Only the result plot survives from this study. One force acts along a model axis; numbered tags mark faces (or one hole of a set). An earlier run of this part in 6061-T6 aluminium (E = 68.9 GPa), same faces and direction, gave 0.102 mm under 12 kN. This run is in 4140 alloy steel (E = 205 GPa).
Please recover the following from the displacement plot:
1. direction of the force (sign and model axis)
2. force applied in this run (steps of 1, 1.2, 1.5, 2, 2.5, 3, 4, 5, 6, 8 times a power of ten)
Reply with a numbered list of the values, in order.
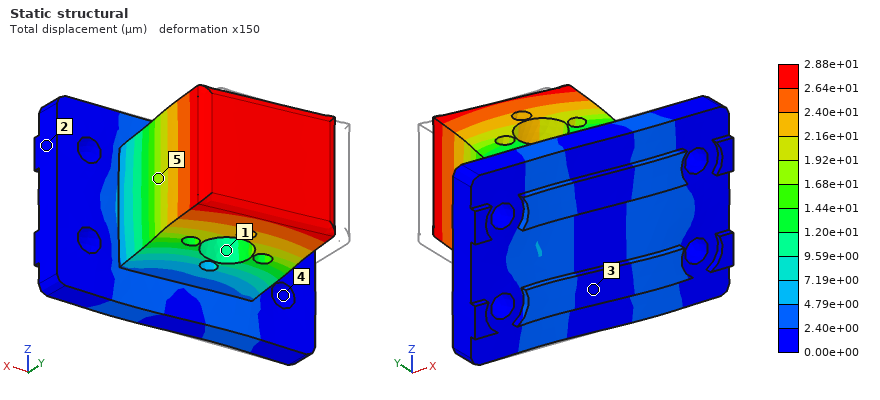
1. +X
2. 10 kN
